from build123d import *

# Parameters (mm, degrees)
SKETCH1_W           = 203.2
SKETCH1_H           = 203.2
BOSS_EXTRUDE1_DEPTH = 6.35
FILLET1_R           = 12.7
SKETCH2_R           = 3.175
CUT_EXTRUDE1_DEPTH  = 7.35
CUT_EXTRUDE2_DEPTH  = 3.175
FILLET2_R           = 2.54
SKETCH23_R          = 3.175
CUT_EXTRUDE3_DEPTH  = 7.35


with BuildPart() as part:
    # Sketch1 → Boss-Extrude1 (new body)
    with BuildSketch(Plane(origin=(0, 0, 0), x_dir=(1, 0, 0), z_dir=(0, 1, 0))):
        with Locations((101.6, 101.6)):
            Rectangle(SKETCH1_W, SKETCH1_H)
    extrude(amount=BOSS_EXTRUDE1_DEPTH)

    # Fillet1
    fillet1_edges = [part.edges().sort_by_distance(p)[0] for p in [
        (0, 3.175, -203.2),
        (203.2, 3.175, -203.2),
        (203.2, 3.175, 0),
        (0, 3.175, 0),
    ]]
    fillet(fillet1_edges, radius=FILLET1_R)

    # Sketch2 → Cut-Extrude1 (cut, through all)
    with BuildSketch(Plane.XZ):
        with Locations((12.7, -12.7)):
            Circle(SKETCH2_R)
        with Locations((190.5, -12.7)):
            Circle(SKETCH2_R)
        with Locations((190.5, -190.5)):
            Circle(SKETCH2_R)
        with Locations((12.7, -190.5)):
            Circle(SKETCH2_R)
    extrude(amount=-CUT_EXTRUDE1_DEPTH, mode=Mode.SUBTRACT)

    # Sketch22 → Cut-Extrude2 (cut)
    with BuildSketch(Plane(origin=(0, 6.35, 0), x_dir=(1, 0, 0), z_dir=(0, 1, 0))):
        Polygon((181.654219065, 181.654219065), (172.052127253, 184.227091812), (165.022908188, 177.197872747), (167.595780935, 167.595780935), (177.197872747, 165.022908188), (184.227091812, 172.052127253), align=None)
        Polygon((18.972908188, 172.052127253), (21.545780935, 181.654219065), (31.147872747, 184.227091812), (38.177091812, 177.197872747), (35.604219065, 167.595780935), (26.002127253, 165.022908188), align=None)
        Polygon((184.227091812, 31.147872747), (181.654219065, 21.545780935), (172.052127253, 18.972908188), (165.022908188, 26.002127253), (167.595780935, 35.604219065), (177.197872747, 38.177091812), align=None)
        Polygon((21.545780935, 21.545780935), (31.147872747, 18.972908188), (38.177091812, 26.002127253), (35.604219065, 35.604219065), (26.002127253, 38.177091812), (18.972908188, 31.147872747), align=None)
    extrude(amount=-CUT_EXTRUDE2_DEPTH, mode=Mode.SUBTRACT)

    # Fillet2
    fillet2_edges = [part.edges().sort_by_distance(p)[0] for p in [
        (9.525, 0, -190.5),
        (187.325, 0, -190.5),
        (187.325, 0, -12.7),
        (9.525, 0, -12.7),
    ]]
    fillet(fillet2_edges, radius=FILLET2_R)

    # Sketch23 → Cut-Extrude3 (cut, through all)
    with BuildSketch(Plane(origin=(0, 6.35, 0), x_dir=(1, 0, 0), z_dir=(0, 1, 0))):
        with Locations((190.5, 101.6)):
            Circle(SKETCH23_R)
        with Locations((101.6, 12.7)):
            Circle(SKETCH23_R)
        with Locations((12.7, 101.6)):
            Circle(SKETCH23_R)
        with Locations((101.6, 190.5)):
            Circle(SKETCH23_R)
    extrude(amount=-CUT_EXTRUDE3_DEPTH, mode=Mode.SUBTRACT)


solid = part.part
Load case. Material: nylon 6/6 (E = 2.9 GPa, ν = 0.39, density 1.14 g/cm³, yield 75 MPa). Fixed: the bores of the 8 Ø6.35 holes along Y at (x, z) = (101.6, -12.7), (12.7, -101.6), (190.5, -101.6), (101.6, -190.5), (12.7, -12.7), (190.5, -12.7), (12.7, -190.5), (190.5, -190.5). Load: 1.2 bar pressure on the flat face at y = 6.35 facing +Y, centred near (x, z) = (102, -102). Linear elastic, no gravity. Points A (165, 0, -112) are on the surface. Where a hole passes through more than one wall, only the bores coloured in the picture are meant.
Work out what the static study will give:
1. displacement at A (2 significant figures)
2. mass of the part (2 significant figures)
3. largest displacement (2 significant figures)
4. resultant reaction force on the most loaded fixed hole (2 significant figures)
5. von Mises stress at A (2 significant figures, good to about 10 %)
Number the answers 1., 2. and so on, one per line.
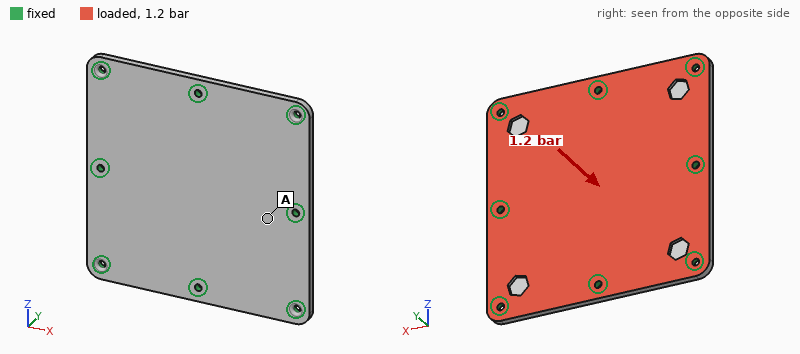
1. 1.1 mm
2. 290 g
3. 3.1 mm
4. 910 N
5. 6.7 MPa
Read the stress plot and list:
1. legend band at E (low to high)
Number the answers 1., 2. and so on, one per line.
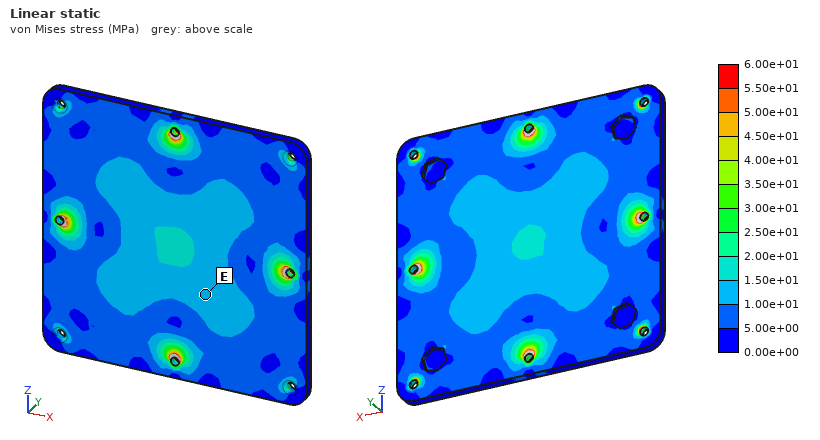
1. 1.00e+01 to 1.50e+01 MPa
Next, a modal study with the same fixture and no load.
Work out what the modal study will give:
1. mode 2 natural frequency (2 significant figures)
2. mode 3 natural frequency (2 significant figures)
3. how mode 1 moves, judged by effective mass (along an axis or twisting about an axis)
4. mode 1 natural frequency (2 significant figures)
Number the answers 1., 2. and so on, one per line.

1. 830 Hz
2. 830 Hz
3. along Y
4. 460 Hz
